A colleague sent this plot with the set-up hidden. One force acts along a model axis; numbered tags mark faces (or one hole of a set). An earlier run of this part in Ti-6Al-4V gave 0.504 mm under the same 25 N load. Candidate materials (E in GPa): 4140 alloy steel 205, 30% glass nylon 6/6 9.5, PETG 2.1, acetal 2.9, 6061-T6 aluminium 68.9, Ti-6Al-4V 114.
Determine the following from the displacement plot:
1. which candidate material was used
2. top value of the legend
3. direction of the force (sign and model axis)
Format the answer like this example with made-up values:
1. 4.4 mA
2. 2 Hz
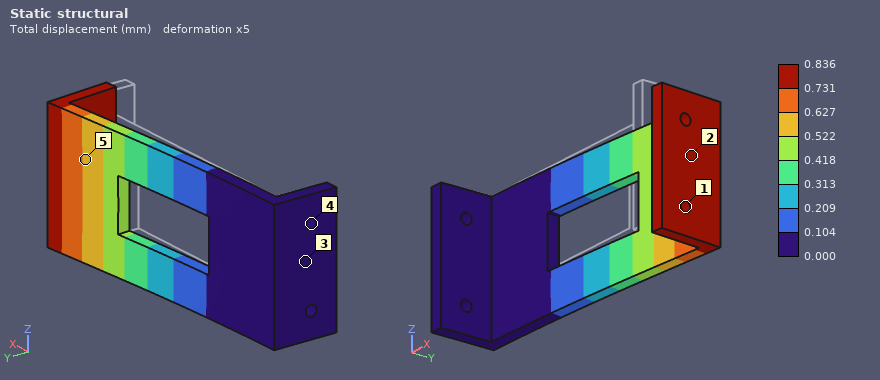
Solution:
1. 6061-T6 aluminium
2. 0.836 mm
3. +Y
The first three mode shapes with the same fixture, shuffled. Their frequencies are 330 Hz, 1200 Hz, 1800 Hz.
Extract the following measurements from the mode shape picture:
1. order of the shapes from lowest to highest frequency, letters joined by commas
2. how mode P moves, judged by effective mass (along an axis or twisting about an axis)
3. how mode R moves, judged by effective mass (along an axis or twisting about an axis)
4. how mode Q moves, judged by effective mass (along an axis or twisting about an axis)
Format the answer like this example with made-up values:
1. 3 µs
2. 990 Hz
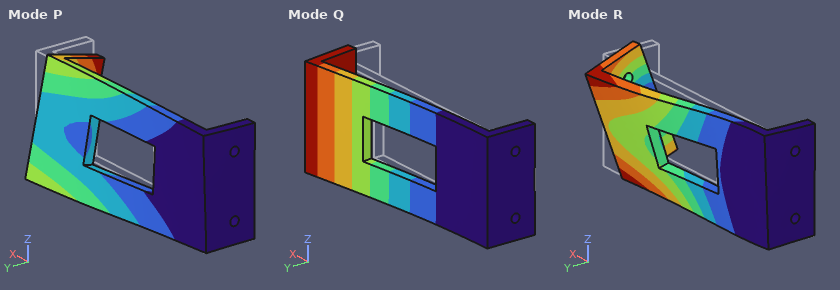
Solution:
1. Q, P, R
2. along Z
3. along Z
4. along Y
